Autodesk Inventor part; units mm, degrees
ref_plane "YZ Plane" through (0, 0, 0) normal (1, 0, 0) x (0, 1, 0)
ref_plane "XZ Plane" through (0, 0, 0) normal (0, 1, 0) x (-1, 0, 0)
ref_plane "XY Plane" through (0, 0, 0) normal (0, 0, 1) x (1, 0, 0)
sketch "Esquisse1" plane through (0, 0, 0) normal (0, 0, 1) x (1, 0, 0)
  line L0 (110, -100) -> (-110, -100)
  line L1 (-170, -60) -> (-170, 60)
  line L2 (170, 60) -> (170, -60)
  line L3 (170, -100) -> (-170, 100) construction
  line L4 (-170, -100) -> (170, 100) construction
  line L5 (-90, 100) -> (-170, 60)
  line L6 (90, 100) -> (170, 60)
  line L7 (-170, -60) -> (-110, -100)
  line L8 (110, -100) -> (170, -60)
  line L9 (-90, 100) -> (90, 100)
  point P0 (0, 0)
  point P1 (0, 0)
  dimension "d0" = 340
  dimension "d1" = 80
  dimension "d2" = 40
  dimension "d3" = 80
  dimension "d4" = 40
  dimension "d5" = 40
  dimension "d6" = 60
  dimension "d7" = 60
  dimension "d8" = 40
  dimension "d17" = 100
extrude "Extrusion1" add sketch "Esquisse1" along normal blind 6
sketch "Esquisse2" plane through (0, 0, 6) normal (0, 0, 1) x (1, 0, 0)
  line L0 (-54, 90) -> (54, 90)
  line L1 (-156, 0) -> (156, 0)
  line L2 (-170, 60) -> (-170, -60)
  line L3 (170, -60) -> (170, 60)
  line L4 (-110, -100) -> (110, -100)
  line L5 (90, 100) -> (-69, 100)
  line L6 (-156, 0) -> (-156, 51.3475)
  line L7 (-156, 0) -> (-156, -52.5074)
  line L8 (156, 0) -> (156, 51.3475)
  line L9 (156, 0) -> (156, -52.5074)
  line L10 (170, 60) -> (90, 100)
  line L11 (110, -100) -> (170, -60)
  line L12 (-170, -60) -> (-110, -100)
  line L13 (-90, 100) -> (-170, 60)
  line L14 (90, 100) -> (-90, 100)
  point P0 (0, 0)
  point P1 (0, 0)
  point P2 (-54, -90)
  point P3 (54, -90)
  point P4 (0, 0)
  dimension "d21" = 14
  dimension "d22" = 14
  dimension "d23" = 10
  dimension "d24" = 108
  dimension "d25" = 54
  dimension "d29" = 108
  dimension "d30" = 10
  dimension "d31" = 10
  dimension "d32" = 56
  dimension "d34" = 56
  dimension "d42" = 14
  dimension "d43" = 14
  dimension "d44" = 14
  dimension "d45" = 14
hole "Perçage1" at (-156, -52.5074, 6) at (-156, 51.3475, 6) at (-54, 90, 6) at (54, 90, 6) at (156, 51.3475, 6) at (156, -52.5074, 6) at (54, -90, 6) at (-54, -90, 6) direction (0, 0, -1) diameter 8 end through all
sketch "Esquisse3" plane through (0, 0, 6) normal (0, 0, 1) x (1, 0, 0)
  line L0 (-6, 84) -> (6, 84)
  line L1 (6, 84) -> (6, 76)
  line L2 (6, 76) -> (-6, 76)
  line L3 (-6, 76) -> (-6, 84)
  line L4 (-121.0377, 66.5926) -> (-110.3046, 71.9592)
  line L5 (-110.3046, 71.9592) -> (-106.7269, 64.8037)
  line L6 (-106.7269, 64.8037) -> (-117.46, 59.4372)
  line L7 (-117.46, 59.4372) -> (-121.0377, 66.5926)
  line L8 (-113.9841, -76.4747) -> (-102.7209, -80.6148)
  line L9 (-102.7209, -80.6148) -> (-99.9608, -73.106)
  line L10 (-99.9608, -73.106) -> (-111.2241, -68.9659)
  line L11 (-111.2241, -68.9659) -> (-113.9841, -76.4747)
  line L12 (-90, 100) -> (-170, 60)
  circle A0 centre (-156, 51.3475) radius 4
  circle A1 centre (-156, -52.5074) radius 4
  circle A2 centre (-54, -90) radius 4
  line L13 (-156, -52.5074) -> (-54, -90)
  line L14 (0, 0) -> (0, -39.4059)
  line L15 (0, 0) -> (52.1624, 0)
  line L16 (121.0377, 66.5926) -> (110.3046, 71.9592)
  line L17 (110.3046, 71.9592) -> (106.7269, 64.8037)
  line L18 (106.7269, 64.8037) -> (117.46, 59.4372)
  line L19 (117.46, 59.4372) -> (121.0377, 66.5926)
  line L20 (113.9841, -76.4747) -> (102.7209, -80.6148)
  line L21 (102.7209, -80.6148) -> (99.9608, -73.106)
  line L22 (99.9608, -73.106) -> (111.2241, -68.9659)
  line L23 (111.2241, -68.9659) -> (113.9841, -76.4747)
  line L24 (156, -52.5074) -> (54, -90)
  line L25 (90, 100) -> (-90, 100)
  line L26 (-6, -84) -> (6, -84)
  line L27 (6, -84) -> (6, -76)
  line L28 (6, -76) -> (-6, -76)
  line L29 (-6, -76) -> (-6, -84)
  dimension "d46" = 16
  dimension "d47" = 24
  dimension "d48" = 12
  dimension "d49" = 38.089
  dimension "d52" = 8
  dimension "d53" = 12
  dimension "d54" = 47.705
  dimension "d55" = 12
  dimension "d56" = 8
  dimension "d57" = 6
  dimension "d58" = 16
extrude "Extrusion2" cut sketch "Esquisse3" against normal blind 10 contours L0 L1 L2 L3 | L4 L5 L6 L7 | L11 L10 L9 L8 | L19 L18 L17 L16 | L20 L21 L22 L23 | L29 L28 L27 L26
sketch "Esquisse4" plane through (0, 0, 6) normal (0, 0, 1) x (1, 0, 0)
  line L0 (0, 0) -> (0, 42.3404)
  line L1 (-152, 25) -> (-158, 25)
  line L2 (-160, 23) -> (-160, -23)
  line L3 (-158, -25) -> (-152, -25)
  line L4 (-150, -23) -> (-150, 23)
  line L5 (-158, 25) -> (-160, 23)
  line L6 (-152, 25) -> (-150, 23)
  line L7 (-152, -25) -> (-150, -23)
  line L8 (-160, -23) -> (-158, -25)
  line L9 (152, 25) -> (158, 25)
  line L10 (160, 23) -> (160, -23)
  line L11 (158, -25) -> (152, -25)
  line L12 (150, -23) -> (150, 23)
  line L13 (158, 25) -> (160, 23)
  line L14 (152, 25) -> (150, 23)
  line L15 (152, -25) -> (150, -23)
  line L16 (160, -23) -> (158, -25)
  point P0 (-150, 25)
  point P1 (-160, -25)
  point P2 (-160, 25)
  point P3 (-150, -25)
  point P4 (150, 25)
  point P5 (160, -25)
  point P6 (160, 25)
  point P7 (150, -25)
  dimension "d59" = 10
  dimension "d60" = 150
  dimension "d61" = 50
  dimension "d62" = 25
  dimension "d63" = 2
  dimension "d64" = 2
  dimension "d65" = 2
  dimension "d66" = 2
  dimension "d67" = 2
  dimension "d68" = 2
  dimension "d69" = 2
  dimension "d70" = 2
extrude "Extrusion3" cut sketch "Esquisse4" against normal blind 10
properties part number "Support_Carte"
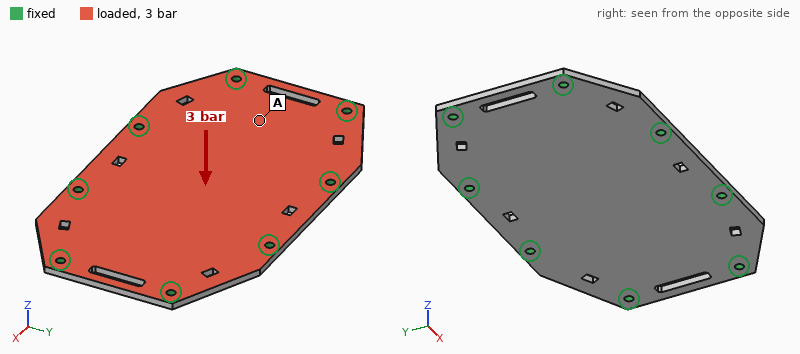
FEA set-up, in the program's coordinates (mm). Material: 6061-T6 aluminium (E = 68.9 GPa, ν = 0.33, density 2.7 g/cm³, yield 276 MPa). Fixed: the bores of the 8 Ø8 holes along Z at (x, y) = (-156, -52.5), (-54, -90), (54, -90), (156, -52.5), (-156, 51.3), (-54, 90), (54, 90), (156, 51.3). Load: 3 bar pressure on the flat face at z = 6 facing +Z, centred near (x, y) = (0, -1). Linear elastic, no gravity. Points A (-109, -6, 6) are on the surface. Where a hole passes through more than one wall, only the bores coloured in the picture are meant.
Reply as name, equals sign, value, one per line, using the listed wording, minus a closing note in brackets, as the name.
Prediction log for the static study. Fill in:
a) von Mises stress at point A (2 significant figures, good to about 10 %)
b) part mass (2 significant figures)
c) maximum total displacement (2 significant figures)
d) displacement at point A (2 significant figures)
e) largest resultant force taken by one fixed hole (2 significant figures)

von Mises stress at point A = 41 MPa
part mass = 980 g
maximum total displacement = 0.87 mm
displacement at point A = 0.43 mm
largest resultant force taken by one fixed hole = 2.9 kN
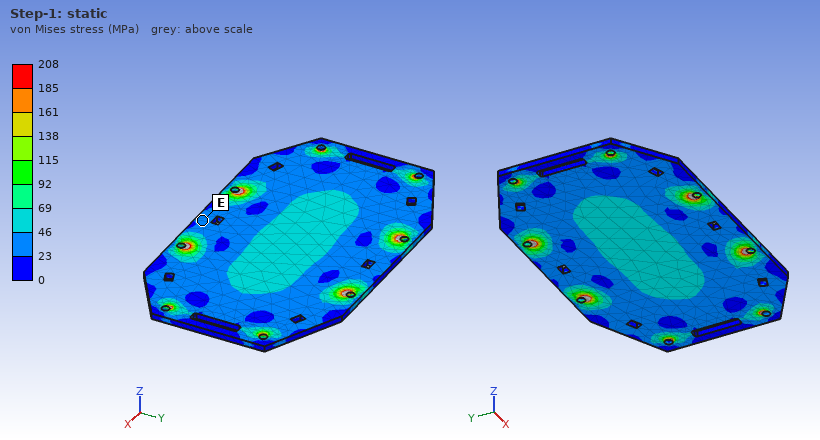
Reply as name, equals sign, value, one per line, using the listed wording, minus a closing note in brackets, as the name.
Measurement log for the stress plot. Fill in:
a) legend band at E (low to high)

legend band at E = 23 to 46 MPa
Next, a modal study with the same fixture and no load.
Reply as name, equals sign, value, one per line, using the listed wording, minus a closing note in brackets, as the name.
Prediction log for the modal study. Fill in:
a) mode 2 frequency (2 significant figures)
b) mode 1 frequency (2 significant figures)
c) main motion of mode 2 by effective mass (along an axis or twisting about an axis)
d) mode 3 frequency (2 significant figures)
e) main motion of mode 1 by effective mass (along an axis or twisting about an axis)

mode 2 frequency = 1300 Hz
mode 1 frequency = 910 Hz
main motion of mode 2 by effective mass = twisting about Y
mode 3 frequency = 1800 Hz
main motion of mode 1 by effective mass = along Z
